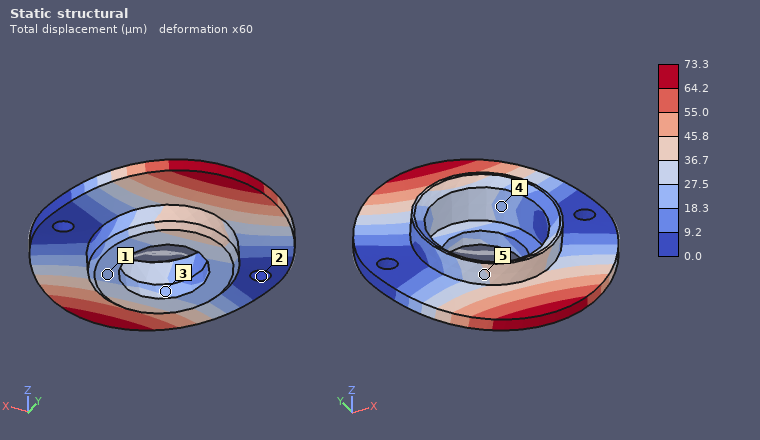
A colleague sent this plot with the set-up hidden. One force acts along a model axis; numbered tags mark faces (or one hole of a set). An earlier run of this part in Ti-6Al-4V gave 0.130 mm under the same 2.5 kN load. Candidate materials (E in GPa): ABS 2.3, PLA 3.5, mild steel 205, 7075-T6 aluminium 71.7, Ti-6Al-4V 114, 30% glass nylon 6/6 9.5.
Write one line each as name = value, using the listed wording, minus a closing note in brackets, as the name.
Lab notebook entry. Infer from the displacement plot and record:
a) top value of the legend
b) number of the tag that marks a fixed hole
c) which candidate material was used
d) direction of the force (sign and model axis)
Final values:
top value of the legend = 73.3 µm
number of the tag that marks a fixed hole = 2
which candidate material was used = mild steel
direction of the force = +Y
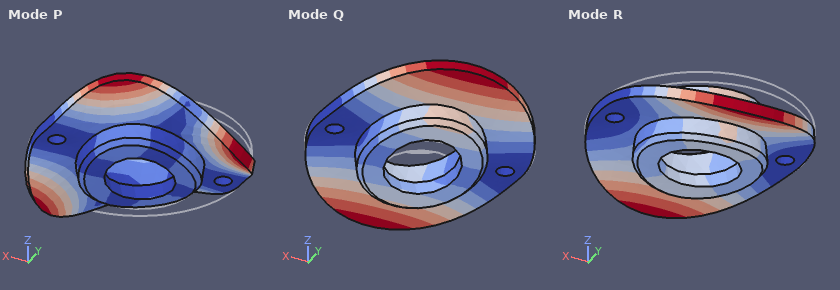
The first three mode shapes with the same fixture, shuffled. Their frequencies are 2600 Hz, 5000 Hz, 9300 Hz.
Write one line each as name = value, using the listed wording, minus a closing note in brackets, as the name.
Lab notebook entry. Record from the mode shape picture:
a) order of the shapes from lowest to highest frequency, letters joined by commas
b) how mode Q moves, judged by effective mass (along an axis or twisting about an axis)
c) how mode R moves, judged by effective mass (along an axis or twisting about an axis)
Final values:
order of the shapes from lowest to highest frequency, letters joined by commas = Q, R, P
how mode Q moves, judged by effective mass = twisting about X
how mode R moves, judged by effective mass = along Z
